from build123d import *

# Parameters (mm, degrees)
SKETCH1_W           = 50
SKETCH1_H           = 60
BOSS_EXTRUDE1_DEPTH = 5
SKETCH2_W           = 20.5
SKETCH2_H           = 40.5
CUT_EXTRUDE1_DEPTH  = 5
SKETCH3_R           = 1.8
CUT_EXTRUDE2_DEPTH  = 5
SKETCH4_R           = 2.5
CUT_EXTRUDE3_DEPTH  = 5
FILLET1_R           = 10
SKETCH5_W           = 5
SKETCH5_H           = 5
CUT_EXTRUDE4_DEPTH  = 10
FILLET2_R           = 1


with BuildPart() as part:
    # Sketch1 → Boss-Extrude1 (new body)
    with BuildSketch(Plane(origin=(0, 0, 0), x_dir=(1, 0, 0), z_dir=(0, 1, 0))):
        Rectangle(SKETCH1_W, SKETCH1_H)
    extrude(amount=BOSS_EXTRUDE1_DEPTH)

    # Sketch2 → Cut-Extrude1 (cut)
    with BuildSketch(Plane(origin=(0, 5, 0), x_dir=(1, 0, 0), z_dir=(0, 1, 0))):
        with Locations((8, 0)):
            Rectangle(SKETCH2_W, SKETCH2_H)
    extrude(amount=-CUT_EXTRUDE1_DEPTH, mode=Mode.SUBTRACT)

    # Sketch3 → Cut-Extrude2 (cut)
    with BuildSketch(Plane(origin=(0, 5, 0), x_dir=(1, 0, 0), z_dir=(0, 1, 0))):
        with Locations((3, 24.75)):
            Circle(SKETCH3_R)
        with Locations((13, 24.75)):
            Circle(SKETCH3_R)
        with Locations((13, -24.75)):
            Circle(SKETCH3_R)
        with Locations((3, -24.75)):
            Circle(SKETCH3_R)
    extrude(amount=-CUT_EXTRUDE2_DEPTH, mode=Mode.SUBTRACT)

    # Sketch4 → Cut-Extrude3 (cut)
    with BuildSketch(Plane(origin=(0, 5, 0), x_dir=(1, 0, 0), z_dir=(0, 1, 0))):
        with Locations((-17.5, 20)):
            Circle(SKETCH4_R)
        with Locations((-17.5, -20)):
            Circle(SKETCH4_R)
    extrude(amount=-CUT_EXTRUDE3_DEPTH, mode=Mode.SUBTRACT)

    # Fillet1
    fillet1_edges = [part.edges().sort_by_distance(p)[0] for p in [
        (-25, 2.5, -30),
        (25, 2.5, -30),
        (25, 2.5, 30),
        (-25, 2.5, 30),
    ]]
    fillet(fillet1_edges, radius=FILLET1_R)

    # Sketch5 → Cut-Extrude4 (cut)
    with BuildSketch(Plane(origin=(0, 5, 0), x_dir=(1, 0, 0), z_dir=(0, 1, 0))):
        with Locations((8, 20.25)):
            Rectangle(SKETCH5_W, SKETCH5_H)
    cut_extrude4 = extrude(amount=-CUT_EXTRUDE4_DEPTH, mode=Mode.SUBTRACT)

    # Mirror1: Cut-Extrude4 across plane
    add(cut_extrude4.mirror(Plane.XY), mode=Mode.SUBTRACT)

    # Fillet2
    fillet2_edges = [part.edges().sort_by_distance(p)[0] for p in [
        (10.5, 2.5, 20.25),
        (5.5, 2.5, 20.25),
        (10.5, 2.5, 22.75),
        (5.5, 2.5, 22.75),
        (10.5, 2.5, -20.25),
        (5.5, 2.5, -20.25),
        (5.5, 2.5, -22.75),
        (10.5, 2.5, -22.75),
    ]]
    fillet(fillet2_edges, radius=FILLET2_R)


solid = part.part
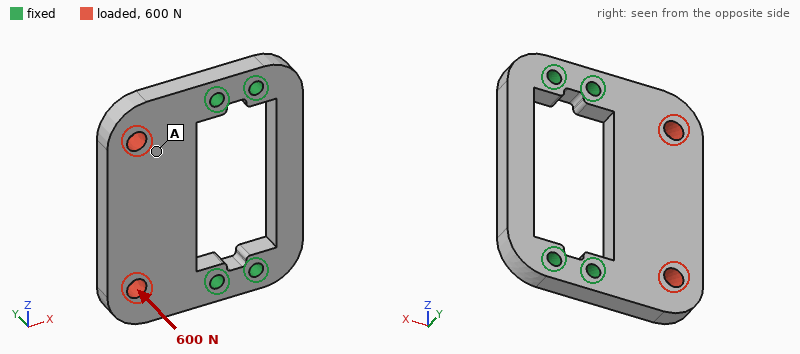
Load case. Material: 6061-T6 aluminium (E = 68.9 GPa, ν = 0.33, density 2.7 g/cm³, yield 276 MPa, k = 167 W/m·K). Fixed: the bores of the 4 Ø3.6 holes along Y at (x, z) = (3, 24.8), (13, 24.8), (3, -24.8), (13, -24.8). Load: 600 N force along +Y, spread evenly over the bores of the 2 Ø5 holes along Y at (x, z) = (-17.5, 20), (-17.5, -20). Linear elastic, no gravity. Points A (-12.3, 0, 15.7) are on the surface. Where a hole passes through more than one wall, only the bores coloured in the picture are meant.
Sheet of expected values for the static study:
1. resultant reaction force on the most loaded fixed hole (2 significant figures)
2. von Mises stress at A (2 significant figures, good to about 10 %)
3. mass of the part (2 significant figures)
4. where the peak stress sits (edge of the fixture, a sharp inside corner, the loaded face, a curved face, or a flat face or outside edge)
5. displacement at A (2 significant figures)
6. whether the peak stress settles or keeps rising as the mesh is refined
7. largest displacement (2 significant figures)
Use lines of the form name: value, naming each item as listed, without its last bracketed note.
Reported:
resultant reaction force on the most loaded fixed hole: 350 N
von Mises stress at A: 16 MPa
mass of the part: 27 g
where the peak stress sits: edge of the fixture
displacement at A: 0.079 mm
whether the peak stress settles or keeps rising as the mesh is refined: keeps rising
largest displacement: 0.18 mm
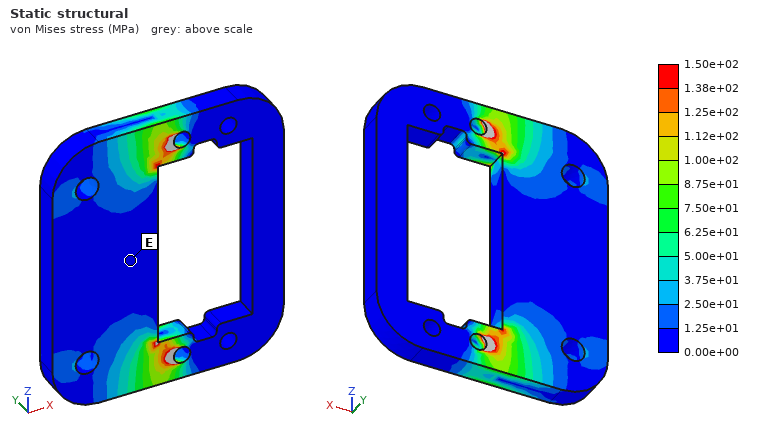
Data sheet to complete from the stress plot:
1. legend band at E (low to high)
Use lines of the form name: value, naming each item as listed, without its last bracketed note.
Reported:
legend band at E: 0.00e+00 to 1.25e+01 MPa
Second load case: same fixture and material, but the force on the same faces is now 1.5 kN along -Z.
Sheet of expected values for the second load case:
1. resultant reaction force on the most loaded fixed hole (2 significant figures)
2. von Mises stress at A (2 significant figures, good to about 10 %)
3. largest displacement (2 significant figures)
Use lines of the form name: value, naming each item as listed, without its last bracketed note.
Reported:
resultant reaction force on the most loaded fixed hole: 920 N
von Mises stress at A: 14 MPa
largest displacement: 15 µm
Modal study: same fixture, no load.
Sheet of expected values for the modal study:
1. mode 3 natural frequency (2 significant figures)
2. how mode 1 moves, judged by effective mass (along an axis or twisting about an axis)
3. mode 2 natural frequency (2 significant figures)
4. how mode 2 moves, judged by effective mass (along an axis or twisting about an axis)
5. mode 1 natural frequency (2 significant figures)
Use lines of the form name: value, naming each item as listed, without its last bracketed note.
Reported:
mode 3 natural frequency: 8100 Hz
how mode 1 moves, judged by effective mass: along Y
mode 2 natural frequency: 7500 Hz
how mode 2 moves, judged by effective mass: twisting about X
mode 1 natural frequency: 3100 Hz
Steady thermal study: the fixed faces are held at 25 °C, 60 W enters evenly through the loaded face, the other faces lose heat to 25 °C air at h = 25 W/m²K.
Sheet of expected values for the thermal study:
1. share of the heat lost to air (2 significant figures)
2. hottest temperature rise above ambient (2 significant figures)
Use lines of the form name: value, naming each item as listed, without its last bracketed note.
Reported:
share of the heat lost to air: 5.8 %
hottest temperature rise above ambient: 56 K
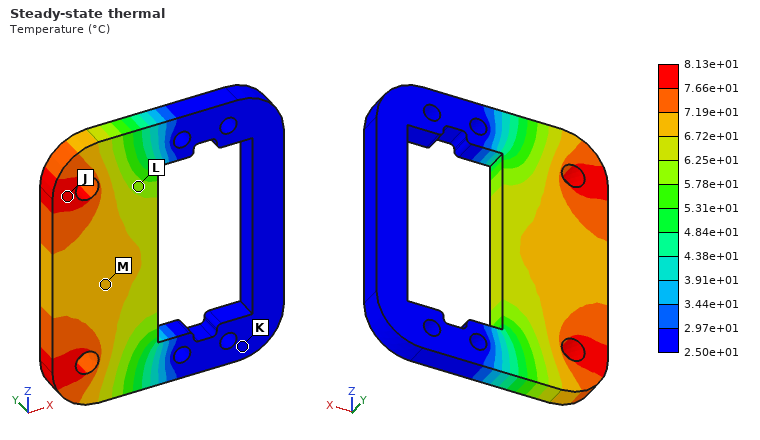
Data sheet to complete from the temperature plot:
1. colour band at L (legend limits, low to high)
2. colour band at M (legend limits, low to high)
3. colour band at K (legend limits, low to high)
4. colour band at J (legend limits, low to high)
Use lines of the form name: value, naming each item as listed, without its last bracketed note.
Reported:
colour band at L: 5.78e+01 to 6.25e+01 °C
colour band at M: 6.72e+01 to 7.19e+01 °C
colour band at K: 2.50e+01 to 2.97e+01 °C
colour band at J: 7.66e+01 to 8.13e+01 °C
